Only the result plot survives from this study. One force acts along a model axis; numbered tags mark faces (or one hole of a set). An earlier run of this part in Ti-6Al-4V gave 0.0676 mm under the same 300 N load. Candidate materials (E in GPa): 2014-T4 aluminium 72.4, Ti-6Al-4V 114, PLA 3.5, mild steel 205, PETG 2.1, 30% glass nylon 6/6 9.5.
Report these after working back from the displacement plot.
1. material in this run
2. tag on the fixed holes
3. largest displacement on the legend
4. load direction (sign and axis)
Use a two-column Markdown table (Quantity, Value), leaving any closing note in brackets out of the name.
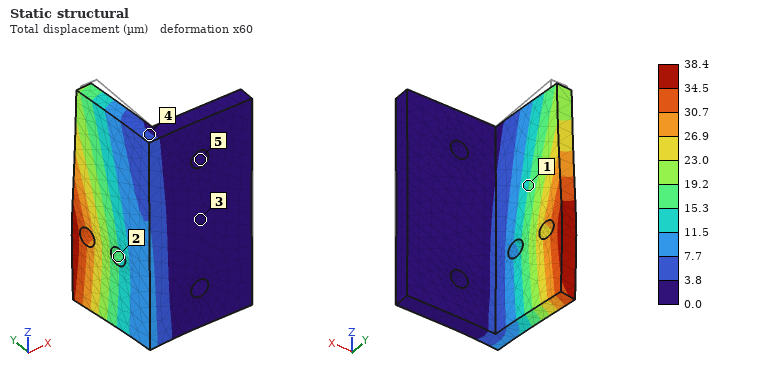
| Quantity | Value |
|---|---|
| material in this run | mild steel |
| tag on the fixed holes | 5 |
| largest displacement on the legend | 38.4 µm |
| load direction | -X |
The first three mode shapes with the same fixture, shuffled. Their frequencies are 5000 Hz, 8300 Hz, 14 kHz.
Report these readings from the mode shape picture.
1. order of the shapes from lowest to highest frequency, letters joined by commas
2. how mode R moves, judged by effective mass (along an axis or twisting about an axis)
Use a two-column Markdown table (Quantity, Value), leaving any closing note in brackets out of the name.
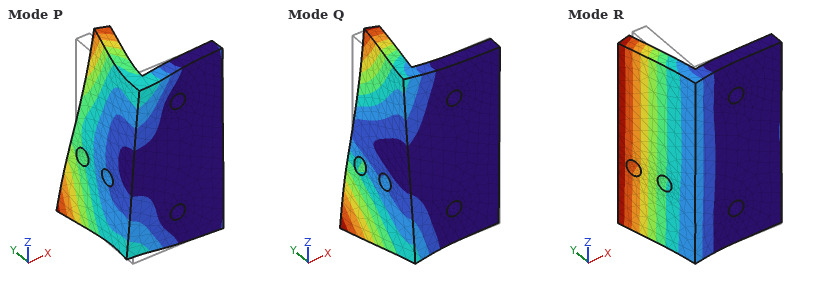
| Quantity | Value |
|---|---|
| order of the shapes from lowest to highest frequency, letters joined by commas | R, Q, P |
| how mode R moves, judged by effective mass | along X |
